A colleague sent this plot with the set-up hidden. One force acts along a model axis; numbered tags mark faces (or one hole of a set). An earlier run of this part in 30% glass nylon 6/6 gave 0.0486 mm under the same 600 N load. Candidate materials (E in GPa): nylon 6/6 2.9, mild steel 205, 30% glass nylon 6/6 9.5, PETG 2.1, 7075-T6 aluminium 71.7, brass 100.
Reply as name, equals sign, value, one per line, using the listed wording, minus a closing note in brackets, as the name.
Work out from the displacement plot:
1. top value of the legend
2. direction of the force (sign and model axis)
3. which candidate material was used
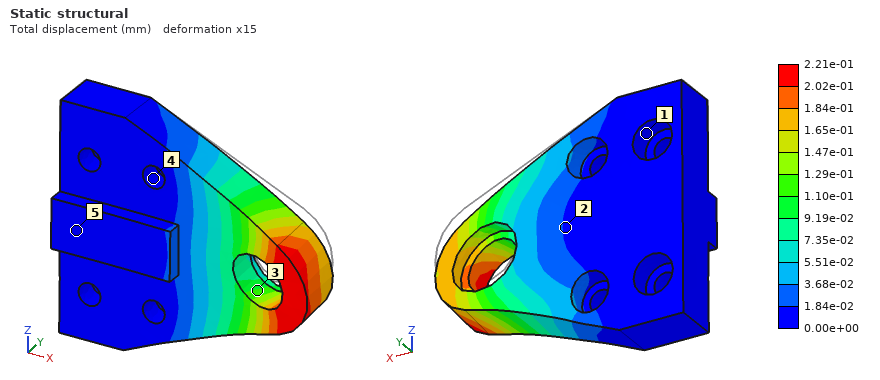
top value of the legend = 2.21e-01 mm
direction of the force = -Z
which candidate material was used = PETG
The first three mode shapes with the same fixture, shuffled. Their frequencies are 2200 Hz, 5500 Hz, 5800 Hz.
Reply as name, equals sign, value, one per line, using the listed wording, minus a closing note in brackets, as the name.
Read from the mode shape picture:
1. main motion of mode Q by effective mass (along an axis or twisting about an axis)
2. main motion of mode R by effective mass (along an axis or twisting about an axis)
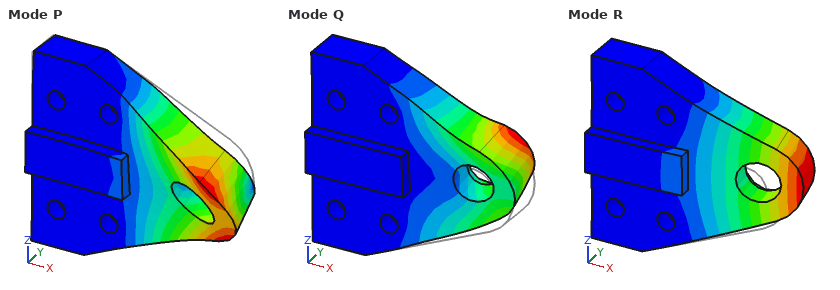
main motion of mode Q by effective mass = along Z
main motion of mode R by effective mass = along Y
